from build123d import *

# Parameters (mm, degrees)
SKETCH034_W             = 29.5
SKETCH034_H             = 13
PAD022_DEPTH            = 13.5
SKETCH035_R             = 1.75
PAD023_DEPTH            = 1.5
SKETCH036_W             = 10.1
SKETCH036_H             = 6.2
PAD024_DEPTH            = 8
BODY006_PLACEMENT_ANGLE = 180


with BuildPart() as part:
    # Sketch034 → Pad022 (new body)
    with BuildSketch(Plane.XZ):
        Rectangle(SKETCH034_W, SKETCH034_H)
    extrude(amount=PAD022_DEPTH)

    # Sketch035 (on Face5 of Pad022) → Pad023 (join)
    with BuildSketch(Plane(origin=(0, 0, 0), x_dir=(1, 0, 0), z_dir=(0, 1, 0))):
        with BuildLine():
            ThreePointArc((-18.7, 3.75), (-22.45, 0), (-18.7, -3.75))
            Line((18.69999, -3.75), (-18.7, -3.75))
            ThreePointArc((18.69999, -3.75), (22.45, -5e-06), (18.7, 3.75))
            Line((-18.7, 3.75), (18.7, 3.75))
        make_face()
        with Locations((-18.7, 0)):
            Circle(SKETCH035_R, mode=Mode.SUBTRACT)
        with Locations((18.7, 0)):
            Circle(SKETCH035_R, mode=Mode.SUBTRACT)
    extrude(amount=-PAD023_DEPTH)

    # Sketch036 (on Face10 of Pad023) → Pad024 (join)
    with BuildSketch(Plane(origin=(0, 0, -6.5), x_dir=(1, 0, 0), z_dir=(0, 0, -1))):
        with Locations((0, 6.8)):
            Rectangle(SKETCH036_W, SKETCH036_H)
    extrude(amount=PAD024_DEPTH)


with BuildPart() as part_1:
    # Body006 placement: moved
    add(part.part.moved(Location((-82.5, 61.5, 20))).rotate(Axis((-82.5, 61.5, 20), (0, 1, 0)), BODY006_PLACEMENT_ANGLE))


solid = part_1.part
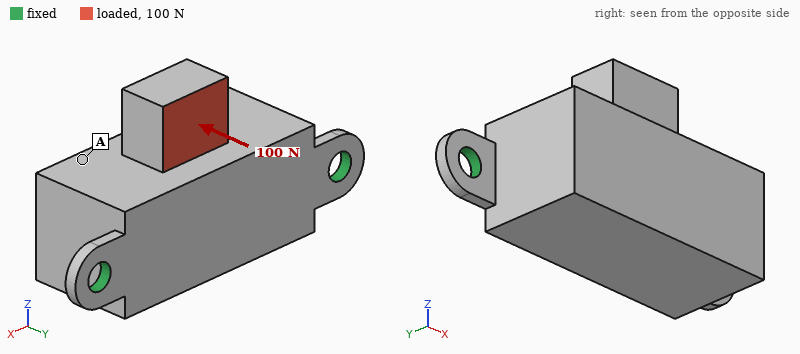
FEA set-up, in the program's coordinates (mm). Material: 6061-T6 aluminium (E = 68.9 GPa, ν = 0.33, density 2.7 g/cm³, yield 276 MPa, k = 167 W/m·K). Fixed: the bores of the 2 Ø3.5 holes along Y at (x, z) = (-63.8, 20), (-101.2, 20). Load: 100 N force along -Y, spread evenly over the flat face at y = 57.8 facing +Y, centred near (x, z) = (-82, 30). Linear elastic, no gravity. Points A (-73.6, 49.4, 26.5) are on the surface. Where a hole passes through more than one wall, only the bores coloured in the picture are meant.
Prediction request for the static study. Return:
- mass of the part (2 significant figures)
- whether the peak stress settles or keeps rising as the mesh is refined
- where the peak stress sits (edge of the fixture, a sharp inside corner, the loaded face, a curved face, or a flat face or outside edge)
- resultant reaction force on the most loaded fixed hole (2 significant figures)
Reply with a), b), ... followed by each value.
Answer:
a) 16 g
b) keeps rising
c) edge of the fixture
d) 62 N
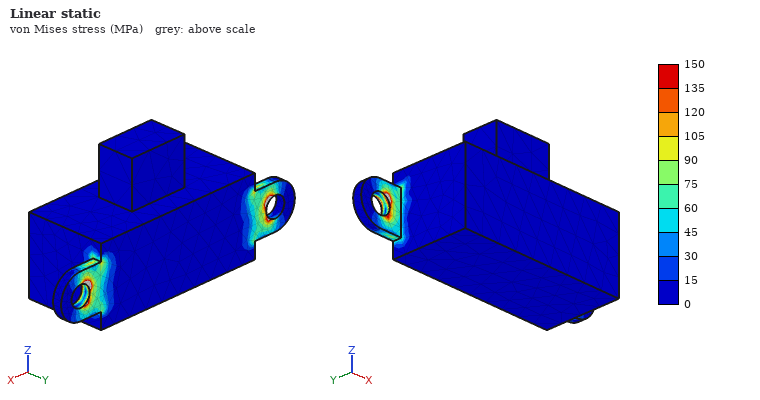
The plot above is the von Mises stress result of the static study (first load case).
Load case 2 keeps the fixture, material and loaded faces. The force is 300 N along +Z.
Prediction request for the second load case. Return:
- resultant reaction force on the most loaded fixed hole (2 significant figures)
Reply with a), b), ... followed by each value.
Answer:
a) 150 N
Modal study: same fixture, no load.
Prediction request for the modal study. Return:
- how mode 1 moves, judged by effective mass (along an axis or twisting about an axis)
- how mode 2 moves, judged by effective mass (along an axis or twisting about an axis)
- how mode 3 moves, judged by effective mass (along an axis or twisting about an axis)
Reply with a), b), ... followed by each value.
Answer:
a) along Z
b) along Y
c) along X
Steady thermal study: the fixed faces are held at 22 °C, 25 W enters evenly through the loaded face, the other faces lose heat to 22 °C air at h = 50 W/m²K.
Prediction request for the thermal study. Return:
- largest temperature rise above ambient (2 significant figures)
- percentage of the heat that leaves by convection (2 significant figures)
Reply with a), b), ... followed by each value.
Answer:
a) 48 K
b) 12 %
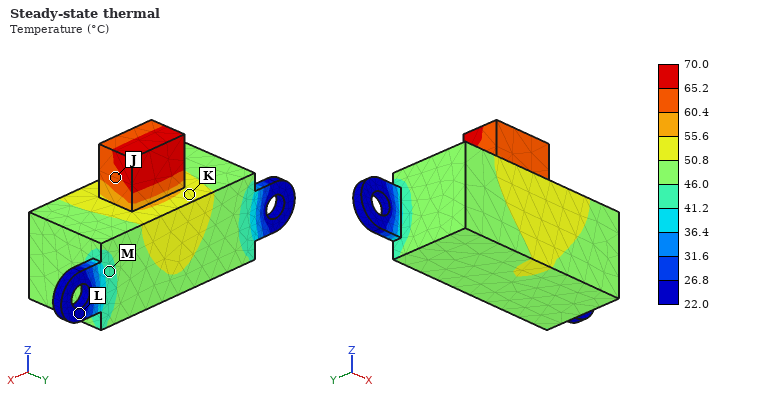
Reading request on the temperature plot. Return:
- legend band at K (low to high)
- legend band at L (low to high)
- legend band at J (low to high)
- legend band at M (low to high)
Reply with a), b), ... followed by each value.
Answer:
a) 50.8 to 55.6 °C
b) 22.0 to 26.8 °C
c) 60.4 to 65.2 °C
d) 41.2 to 46.0 °C
